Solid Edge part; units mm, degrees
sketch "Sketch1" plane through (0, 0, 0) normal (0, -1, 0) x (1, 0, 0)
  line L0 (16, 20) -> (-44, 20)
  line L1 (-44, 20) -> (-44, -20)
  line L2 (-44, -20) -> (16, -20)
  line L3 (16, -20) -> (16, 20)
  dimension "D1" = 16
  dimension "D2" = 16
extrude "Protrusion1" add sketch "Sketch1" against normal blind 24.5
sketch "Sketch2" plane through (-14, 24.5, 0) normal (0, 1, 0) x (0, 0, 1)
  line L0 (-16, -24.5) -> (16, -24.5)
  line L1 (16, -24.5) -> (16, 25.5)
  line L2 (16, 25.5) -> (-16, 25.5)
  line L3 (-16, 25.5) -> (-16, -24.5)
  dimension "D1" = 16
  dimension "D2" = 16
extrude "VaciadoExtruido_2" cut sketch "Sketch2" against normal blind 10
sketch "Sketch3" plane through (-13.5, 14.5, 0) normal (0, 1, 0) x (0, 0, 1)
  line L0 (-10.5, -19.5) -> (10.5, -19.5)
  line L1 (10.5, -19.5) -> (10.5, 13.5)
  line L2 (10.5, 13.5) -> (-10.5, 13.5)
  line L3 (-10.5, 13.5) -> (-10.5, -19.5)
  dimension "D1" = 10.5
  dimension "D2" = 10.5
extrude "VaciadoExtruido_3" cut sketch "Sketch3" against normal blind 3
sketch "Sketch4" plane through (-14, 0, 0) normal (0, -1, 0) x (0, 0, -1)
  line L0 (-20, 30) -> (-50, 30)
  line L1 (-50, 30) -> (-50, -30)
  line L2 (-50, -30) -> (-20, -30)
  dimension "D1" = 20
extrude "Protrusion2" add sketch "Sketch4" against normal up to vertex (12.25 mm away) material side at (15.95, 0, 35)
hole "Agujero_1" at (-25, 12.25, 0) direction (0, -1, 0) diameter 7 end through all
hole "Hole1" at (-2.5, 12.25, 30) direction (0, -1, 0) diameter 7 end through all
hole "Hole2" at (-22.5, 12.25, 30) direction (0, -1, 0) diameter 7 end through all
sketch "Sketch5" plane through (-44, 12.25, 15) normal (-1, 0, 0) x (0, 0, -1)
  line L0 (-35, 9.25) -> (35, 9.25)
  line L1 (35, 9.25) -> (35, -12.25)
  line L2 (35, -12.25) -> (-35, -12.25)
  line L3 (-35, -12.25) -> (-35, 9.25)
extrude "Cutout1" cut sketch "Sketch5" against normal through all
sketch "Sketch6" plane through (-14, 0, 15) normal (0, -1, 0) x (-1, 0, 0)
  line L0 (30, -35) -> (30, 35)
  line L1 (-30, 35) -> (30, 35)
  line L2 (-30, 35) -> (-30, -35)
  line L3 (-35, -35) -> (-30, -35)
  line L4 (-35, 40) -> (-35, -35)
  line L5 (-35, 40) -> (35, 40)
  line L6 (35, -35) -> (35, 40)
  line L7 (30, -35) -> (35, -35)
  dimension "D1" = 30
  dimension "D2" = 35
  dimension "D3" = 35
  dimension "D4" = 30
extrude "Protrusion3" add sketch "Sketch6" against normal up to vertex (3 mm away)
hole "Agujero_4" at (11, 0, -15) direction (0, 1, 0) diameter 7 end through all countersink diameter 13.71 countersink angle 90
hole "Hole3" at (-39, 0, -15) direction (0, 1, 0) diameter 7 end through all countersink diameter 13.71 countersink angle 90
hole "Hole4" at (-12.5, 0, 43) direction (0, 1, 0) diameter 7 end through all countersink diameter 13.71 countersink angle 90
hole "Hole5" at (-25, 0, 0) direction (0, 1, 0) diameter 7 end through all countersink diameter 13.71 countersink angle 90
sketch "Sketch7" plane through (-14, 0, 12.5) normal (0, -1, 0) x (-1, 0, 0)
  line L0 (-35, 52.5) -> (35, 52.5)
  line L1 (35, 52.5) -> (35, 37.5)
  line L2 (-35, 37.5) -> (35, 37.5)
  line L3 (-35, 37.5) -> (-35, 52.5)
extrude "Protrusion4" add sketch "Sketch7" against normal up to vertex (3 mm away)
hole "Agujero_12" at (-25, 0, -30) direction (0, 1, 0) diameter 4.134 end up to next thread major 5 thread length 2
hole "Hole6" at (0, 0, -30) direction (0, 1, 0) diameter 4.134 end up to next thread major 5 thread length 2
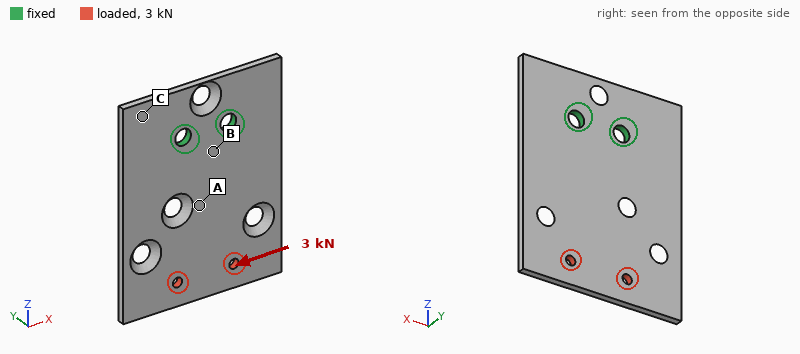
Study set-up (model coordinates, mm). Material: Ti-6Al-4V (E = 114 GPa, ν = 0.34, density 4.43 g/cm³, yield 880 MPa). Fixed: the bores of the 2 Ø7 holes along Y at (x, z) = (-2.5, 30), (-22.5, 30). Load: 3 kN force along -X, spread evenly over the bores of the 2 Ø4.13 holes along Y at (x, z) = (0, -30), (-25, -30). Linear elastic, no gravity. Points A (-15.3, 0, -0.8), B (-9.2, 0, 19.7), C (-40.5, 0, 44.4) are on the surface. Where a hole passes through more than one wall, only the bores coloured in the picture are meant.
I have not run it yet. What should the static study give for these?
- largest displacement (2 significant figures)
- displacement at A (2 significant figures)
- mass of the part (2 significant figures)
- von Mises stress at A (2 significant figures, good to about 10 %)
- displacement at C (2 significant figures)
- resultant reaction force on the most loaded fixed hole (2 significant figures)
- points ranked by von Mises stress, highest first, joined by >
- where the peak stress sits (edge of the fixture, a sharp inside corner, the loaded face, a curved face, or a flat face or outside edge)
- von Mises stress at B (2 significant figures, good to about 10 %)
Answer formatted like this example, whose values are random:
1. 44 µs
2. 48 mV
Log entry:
1. 0.15 mm
2. 0.054 mm
3. 77 g
4. 60 MPa
5. 0.038 mm
6. 6.8 kN
7. B > A > C
8. edge of the fixture
9. 100 MPa
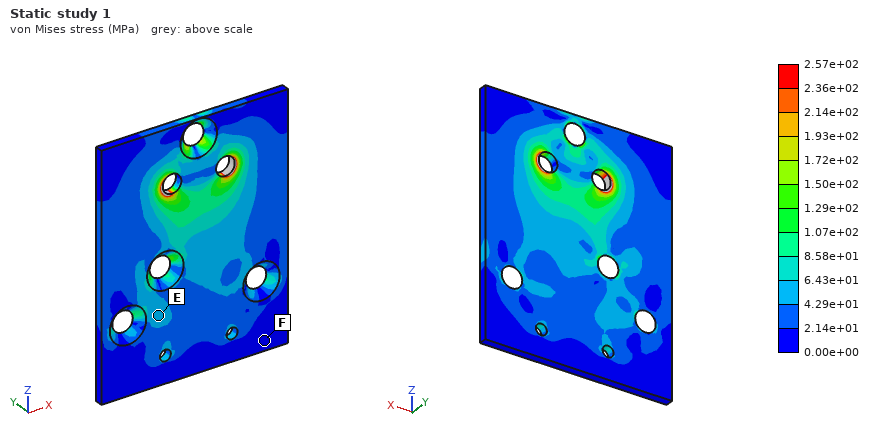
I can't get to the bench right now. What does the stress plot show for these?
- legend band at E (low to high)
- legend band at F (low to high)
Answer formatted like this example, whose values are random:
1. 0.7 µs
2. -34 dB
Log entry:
1. 4.29e+01 to 6.43e+01 MPa
2. 0.00e+00 to 2.14e+01 MPa
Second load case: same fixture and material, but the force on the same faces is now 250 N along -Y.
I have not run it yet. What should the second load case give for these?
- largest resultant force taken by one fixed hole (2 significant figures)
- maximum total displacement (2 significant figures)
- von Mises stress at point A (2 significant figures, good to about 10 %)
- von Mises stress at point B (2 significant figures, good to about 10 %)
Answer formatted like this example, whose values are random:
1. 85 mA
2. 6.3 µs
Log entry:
1. 130 N
2. 1.3 mm
3. 98 MPa
4. 130 MPa
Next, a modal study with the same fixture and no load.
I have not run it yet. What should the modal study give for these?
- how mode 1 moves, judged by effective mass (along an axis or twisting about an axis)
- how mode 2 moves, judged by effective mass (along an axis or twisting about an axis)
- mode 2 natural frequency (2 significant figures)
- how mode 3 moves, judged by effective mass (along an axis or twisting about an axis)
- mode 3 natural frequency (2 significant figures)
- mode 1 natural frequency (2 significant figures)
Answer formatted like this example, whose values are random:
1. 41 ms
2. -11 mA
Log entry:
1. along Y
2. twisting about Z
3. 1100 Hz
4. along Y
5. 2700 Hz
6. 520 Hz
